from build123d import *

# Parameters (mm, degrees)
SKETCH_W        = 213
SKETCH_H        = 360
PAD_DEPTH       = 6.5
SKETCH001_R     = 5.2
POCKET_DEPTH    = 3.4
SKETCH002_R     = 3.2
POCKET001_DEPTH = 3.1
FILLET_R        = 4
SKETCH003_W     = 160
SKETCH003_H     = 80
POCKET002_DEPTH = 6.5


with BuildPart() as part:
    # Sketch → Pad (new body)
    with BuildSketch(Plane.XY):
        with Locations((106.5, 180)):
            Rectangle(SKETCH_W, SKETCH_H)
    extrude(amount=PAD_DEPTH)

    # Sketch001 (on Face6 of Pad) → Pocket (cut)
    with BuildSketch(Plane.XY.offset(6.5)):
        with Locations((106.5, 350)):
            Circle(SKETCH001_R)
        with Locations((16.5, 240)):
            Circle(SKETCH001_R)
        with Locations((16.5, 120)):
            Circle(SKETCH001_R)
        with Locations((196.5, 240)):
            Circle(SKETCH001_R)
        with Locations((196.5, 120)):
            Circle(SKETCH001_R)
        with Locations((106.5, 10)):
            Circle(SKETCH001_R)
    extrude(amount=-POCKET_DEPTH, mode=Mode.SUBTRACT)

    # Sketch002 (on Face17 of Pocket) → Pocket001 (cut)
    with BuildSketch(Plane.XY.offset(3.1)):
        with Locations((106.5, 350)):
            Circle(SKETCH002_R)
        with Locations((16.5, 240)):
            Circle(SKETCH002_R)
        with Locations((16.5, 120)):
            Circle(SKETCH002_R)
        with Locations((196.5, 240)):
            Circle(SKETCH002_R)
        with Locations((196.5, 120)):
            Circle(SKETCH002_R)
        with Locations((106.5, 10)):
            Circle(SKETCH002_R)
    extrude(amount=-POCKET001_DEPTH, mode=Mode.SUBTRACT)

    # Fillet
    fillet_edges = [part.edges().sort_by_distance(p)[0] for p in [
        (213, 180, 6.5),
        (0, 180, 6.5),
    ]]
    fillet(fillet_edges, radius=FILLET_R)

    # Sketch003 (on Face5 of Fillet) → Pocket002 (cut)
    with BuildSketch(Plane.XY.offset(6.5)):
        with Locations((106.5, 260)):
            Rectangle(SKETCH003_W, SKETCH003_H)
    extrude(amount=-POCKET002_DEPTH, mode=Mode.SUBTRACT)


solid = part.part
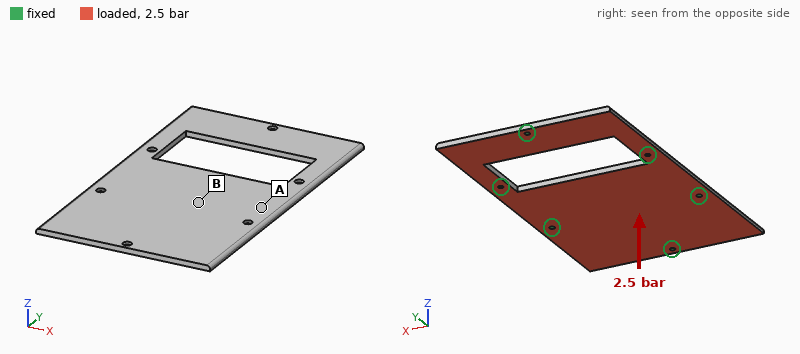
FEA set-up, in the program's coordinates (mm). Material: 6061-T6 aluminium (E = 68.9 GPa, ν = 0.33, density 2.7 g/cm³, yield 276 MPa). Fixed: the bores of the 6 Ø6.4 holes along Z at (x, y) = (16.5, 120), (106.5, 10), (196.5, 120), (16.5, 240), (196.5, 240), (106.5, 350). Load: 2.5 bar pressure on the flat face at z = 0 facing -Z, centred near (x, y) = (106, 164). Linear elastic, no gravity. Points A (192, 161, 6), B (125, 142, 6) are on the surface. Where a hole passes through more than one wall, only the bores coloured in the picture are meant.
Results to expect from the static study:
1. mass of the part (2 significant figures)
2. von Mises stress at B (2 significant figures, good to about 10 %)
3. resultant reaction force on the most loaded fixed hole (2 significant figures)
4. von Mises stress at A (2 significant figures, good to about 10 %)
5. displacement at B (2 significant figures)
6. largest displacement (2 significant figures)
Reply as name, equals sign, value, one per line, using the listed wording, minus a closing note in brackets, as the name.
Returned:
mass of the part = 1.1 kg
von Mises stress at B = 55 MPa
resultant reaction force on the most loaded fixed hole = 5.2 kN
von Mises stress at A = 23 MPa
displacement at B = 0.71 mm
largest displacement = 1.3 mm
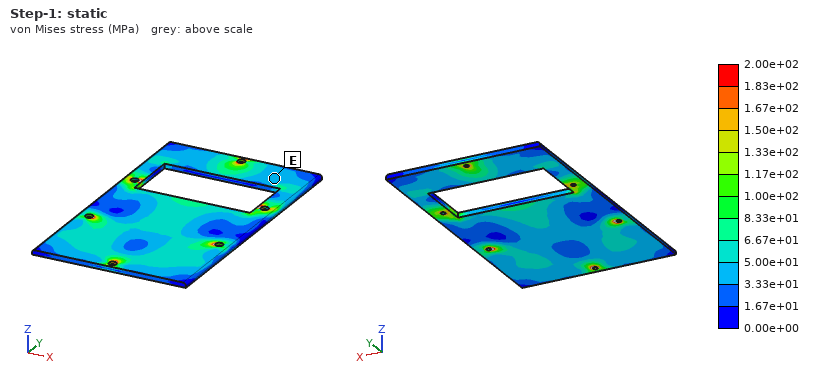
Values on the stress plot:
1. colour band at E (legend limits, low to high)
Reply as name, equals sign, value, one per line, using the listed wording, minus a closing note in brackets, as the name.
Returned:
colour band at E = 3.33e+01 to 5.00e+01 MPa
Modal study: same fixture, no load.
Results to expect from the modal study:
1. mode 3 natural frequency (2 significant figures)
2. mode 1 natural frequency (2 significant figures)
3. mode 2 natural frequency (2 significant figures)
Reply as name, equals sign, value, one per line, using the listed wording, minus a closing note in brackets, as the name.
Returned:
mode 3 natural frequency = 670 Hz
mode 1 natural frequency = 560 Hz
mode 2 natural frequency = 670 Hz
